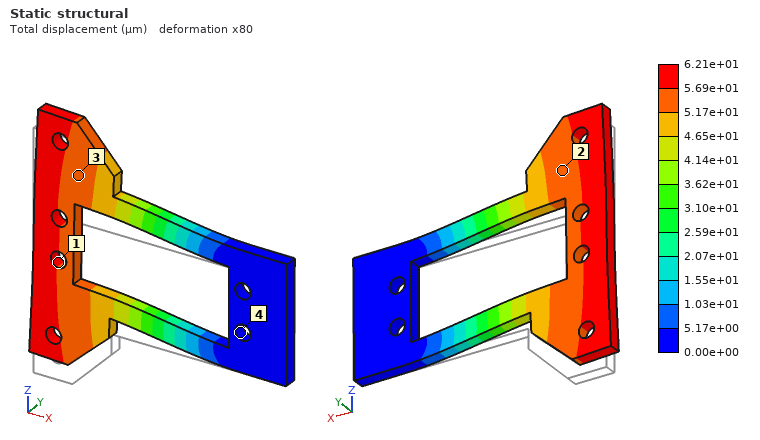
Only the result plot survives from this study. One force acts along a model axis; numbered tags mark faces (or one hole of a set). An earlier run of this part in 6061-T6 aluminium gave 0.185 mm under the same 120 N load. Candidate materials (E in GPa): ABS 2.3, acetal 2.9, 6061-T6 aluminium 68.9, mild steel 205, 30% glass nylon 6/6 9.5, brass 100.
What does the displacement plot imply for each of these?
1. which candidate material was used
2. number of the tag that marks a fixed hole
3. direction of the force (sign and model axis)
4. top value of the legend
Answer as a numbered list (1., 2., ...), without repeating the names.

1. mild steel
2. 4
3. +Z
4. 6.21e+01 µm
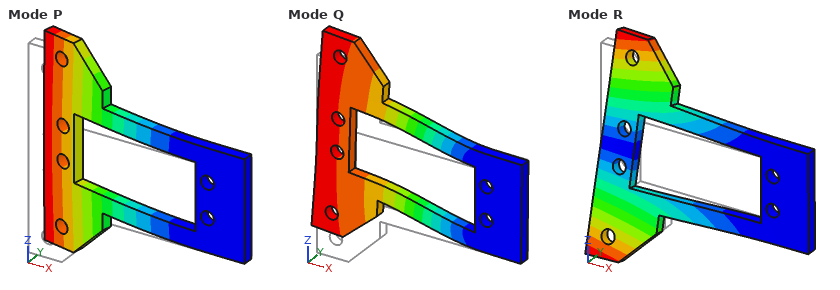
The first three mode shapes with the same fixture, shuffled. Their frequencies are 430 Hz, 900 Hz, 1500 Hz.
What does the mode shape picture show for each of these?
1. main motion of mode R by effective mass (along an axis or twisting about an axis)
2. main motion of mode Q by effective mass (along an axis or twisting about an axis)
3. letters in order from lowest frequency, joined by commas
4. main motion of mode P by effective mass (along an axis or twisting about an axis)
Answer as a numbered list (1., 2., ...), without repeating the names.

1. twisting about X
2. along Z
3. P, R, Q
4. along Y
